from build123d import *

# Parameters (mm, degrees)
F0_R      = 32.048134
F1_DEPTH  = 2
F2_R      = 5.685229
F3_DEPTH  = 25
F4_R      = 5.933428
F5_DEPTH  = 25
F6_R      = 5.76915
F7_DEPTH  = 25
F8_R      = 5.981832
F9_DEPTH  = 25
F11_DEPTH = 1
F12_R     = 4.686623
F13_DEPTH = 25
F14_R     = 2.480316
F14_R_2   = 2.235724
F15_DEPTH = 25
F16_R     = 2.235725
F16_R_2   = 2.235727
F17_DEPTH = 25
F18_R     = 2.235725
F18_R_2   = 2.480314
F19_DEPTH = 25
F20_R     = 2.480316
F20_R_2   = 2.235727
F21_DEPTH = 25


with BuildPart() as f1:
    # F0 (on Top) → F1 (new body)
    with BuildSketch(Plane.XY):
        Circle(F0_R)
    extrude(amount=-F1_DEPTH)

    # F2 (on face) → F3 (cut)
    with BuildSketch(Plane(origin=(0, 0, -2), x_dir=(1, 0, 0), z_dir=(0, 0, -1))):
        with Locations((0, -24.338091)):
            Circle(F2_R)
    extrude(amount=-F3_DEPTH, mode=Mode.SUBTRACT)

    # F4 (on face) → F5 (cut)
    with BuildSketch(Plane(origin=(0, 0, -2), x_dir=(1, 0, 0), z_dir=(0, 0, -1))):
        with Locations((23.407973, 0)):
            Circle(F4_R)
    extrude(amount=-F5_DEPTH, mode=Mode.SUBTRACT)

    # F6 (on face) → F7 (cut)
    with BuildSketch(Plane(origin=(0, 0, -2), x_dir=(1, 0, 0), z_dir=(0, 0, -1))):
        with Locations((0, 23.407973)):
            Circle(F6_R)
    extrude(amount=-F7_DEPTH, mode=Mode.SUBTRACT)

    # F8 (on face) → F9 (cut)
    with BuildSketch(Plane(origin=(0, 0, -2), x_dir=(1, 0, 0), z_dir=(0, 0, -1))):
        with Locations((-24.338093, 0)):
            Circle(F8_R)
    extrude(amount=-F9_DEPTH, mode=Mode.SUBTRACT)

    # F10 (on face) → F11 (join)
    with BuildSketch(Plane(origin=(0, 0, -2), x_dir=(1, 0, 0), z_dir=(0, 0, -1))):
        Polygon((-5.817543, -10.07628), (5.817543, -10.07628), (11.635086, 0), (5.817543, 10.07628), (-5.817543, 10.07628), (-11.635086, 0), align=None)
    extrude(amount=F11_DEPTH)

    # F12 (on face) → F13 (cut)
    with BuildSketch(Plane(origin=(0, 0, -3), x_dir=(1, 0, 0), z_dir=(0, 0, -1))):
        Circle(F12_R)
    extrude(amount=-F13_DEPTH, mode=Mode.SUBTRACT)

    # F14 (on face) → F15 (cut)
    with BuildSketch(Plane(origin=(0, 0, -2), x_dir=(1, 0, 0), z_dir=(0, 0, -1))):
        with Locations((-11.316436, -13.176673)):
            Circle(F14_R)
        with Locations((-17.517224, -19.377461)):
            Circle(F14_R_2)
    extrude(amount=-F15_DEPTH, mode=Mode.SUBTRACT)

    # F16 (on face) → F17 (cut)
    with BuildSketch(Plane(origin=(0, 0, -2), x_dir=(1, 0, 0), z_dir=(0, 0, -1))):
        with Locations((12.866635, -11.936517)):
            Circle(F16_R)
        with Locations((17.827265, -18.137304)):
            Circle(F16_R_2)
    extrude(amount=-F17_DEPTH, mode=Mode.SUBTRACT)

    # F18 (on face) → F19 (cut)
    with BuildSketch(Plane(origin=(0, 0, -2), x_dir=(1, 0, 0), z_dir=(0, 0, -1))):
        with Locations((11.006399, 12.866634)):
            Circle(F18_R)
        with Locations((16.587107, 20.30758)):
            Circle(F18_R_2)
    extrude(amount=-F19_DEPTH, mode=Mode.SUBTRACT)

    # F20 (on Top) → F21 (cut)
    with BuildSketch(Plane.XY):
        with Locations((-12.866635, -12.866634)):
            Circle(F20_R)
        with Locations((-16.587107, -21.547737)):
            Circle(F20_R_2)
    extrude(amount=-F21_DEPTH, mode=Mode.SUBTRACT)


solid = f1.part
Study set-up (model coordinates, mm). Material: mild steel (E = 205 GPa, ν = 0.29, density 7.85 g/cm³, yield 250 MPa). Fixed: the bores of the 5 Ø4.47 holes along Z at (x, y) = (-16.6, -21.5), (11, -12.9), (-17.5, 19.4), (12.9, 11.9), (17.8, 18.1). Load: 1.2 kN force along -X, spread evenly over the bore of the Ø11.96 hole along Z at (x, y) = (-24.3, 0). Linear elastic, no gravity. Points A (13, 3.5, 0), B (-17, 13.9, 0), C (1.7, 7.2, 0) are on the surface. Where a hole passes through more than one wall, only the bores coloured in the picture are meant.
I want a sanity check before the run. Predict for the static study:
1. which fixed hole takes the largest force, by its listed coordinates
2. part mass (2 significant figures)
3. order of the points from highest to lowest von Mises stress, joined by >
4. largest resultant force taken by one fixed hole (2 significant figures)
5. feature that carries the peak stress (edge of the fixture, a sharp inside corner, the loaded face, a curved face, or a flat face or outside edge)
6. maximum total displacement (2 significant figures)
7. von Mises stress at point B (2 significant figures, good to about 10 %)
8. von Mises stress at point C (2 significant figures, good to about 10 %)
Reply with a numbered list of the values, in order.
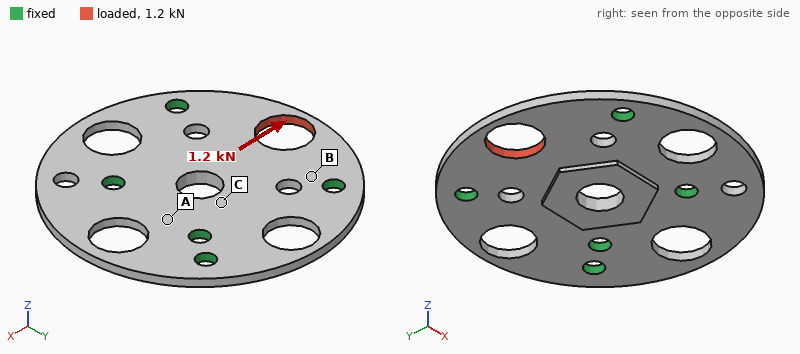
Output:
1. (-17.5, 19.4)
2. 43 g
3. B > C > A
4. 370 N
5. a curved face
6. 7.0 µm
7. 25 MPa
8. 16 MPa
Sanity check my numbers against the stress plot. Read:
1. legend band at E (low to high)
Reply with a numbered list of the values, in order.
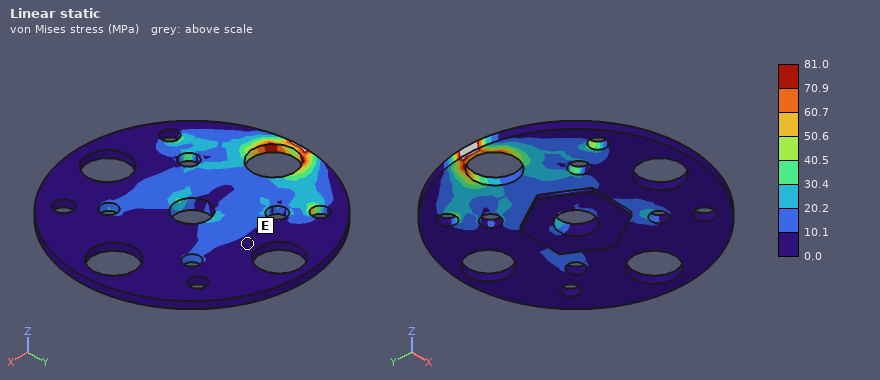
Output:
1. 0.0 to 10.1 MPa
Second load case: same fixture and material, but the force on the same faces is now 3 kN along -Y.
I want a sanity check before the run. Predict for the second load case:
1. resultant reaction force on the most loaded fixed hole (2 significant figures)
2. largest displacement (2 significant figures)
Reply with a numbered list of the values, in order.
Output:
1. 1.6 kN
2. 12 µm
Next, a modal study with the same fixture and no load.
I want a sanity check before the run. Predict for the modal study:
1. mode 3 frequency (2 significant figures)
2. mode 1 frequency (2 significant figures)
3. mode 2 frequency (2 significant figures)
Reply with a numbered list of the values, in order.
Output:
1. 7100 Hz
2. 5900 Hz
3. 6000 Hz
